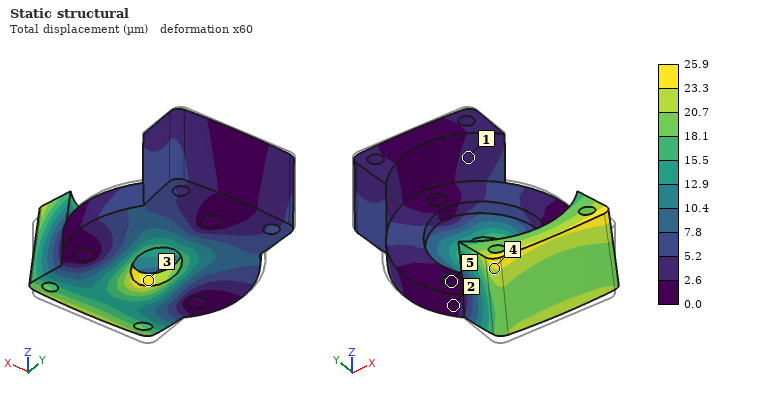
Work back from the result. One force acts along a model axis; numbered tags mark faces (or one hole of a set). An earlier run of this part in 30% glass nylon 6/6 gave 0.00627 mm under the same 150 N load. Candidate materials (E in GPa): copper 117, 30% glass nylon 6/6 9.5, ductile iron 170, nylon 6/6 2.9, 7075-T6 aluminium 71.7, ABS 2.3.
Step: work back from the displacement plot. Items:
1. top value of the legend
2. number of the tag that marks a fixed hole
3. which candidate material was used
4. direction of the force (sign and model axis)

25.9 µm
5
ABS
-Y
